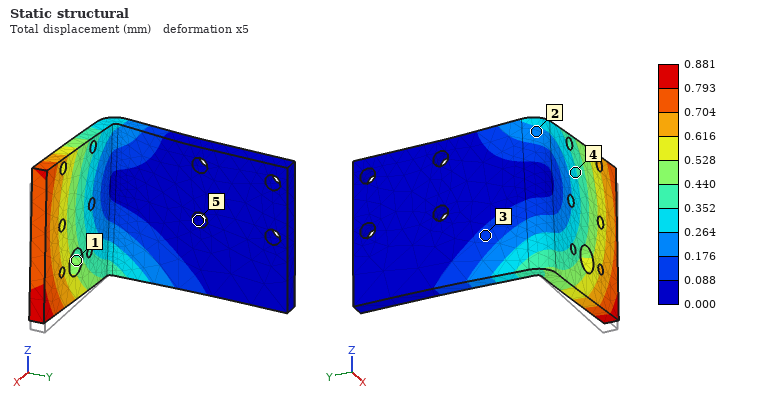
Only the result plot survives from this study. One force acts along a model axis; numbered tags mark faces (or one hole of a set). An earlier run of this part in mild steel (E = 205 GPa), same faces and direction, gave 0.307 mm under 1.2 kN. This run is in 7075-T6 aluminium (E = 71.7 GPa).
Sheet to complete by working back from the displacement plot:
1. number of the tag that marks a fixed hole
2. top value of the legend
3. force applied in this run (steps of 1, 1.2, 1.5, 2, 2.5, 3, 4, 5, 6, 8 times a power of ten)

5
0.881 mm
1.2 kN
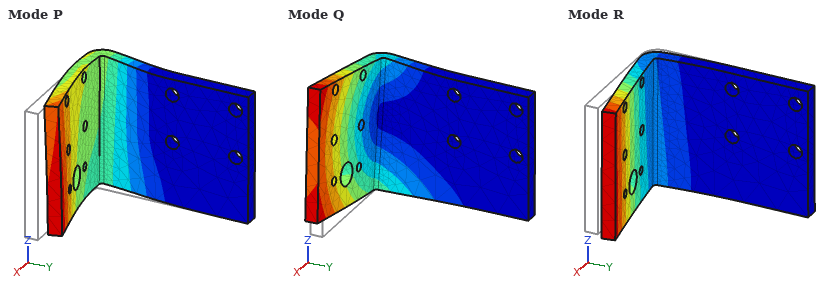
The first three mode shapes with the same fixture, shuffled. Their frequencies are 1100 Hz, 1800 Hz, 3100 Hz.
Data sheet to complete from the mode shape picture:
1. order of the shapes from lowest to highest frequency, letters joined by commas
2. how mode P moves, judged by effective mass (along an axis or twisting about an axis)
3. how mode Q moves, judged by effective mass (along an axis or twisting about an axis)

R, Q, P
along X
along Z
